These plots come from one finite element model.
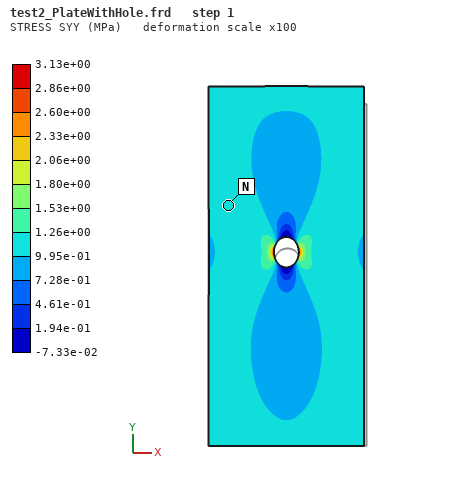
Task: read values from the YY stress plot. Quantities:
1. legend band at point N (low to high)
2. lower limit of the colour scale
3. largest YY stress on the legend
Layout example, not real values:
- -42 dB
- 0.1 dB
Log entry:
- 9.95e-01 to 1.26e+00 MPa
- -7.33e-02 MPa
- 3.13e+00 MPa
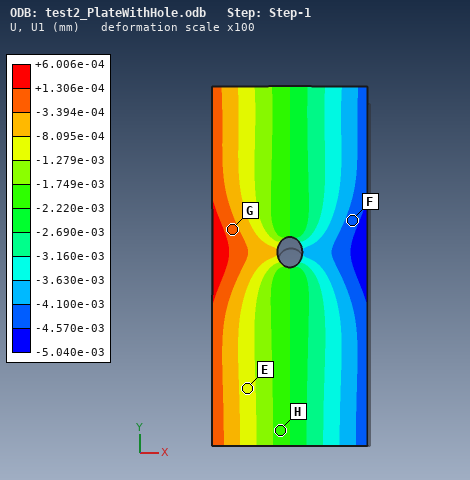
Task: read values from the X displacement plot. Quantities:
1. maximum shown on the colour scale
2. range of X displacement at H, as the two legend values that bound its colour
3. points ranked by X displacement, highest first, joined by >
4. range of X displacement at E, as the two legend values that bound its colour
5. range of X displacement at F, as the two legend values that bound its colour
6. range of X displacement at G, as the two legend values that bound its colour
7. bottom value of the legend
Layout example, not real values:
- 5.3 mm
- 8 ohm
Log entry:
- +6.006e-04 mm
- -2.220e-03 to -1.749e-03 mm
- G > E > H > F
- -1.279e-03 to -8.095e-04 mm
- -4.570e-03 to -4.100e-03 mm
- -3.394e-04 to +1.306e-04 mm
- -5.040e-03 mm
